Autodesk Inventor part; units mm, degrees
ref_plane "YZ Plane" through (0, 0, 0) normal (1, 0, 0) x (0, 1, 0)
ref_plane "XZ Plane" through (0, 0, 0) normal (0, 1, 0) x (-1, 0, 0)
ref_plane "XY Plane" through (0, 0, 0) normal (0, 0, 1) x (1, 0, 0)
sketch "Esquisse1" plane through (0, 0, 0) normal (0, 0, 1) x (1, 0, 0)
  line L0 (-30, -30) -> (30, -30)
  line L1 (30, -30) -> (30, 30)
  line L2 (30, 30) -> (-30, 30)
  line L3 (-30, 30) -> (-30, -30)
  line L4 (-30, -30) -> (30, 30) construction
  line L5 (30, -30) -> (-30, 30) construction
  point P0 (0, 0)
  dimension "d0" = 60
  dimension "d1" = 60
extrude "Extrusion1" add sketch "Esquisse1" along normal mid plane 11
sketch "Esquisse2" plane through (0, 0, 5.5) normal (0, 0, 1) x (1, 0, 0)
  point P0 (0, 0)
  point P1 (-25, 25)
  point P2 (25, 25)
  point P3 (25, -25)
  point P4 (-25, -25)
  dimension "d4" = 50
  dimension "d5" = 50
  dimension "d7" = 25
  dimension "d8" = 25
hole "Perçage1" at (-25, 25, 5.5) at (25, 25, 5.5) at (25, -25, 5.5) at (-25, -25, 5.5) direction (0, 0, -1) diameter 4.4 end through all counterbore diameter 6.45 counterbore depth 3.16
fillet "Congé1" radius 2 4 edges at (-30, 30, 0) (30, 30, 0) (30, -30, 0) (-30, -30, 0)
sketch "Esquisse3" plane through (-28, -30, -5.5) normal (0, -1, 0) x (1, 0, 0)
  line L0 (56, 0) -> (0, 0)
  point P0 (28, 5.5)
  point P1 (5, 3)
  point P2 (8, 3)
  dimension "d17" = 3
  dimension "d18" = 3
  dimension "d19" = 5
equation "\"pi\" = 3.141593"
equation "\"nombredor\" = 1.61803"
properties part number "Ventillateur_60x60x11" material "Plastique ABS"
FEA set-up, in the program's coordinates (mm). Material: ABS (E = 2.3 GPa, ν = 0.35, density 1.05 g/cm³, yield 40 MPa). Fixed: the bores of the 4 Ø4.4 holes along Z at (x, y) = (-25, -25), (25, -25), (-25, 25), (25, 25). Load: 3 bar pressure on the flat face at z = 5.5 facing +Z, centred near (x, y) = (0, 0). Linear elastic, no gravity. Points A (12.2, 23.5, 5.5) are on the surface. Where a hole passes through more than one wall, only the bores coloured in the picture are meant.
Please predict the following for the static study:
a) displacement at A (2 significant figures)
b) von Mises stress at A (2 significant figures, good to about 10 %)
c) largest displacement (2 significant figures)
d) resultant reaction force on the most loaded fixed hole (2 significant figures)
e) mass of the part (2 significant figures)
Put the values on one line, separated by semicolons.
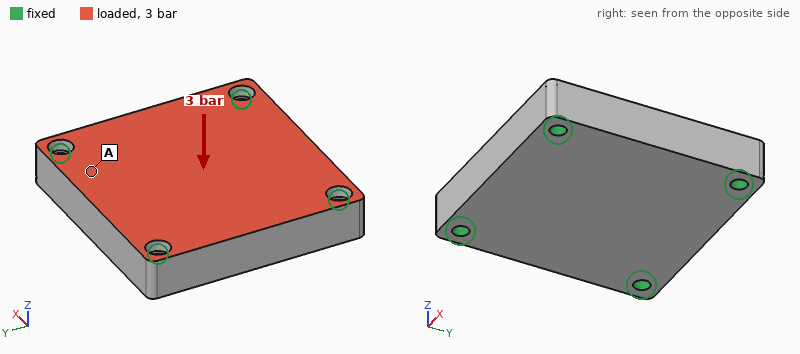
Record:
46 µm; 1.7 MPa; 87 µm; 280 N; 41 g
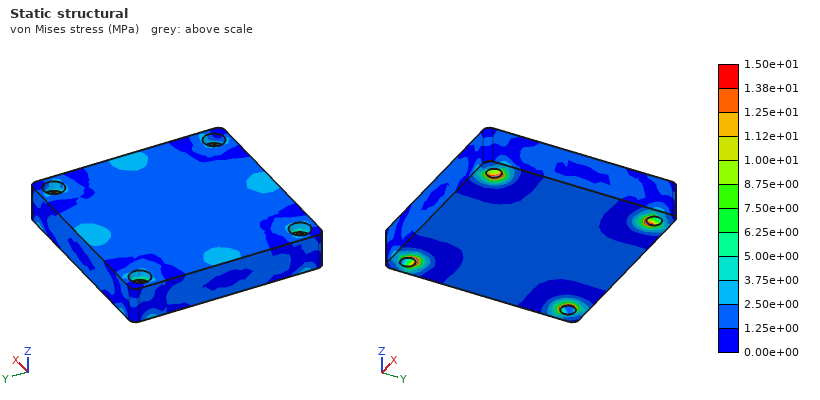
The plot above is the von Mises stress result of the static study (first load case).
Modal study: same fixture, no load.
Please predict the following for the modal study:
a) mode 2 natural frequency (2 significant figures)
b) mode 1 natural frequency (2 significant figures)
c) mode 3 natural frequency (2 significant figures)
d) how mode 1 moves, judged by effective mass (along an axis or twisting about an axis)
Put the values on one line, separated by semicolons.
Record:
5100 Hz; 3200 Hz; 5100 Hz; along Z
